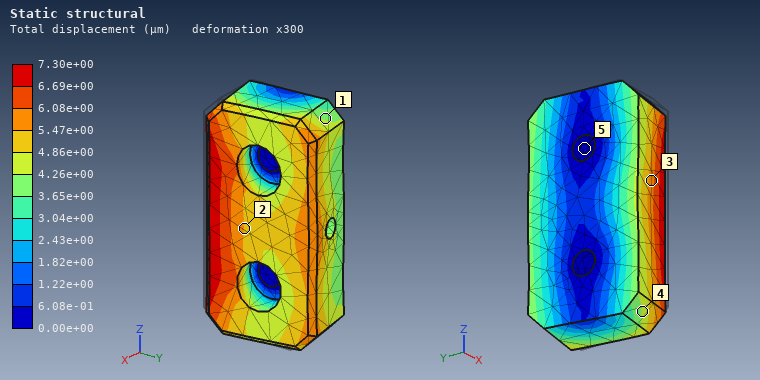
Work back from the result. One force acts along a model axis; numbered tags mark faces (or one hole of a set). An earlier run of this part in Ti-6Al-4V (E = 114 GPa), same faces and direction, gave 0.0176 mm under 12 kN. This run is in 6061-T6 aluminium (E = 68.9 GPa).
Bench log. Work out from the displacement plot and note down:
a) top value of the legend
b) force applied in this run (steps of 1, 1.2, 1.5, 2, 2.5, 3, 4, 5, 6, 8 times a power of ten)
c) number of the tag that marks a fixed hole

7.30e+00 µm
3 kN
5
